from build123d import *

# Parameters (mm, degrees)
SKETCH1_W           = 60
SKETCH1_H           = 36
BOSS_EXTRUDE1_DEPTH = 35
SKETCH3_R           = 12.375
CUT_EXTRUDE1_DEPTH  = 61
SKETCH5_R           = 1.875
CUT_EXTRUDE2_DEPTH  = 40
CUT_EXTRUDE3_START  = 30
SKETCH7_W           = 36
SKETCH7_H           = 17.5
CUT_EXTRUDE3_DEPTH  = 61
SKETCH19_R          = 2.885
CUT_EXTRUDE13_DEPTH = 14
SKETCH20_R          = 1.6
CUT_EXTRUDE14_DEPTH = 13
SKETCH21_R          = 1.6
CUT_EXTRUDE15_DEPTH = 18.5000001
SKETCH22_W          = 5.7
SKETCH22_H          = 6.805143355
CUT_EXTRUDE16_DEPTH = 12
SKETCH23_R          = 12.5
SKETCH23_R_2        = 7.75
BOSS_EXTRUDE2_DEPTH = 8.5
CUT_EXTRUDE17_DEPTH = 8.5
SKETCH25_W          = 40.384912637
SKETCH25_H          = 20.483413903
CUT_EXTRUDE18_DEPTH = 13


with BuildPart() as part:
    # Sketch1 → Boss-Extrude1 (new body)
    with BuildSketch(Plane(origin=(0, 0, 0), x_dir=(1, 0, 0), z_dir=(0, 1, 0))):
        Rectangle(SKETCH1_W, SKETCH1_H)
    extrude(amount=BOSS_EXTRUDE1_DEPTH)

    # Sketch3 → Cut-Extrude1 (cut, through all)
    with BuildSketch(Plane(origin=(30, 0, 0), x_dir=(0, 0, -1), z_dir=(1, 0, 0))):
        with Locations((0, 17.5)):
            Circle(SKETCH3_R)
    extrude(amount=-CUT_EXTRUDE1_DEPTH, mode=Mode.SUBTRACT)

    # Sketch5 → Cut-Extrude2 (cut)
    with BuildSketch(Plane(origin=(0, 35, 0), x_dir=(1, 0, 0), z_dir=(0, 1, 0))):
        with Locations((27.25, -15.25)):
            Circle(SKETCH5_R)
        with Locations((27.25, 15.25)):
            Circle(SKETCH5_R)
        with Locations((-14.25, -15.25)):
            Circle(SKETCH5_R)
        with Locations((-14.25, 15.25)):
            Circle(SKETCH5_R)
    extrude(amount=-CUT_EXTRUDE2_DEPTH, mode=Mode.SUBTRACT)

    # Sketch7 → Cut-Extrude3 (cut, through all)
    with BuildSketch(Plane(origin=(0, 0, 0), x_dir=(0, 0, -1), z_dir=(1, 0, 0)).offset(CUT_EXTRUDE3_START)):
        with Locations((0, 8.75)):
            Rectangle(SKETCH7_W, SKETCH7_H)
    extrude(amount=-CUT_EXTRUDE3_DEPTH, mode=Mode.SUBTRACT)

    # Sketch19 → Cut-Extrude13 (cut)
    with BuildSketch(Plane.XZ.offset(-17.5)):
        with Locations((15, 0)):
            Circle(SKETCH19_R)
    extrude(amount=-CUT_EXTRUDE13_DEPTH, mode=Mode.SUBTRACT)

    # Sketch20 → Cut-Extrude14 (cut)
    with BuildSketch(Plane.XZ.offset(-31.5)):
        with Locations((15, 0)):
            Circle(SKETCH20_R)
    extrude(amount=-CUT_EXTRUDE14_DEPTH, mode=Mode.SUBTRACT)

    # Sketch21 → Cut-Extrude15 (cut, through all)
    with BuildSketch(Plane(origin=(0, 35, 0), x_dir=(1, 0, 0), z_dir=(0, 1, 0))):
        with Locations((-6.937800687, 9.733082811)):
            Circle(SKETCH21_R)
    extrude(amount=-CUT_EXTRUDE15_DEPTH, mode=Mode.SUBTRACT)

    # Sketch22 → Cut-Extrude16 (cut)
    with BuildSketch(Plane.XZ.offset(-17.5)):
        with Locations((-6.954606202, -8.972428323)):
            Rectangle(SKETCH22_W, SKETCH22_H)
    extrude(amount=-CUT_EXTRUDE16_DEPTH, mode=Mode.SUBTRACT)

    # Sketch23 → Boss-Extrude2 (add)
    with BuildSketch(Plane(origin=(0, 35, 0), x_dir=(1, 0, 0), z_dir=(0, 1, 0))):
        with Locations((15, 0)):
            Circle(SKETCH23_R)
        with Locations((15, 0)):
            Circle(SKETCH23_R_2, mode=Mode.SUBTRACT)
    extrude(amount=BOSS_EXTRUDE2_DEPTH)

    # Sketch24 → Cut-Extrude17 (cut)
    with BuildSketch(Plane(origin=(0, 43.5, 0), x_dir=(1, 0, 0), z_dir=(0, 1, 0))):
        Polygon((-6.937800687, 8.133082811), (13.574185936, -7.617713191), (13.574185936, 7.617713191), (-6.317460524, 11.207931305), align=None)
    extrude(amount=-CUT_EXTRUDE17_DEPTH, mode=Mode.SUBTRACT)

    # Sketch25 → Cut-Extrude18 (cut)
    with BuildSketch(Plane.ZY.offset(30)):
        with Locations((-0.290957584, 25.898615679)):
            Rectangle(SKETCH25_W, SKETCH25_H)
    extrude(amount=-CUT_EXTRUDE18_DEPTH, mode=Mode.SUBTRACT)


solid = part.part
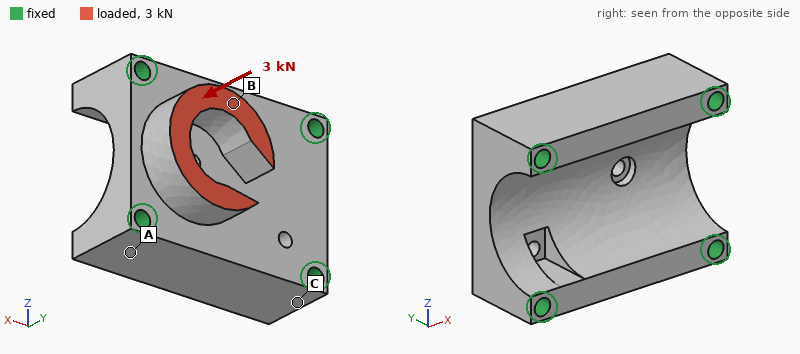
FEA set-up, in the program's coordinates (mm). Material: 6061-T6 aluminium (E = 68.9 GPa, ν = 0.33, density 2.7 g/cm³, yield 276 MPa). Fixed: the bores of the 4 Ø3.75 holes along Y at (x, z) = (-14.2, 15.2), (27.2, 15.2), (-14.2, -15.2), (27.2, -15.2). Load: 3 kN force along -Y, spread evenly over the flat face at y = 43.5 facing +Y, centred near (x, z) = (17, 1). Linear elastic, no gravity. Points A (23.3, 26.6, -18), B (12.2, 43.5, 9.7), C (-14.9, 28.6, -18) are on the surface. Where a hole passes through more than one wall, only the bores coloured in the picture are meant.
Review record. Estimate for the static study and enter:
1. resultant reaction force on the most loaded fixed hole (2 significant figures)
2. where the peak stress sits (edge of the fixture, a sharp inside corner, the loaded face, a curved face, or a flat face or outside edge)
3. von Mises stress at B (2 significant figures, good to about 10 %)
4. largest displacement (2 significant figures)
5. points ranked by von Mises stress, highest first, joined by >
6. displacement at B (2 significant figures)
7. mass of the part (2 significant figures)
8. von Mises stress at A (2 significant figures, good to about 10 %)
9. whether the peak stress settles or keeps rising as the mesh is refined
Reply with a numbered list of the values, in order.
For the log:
1. 1.3 kN
2. edge of the fixture
3. 11 MPa
4. 8.1 µm
5. B > A > C
6. 6.0 µm
7. 52 g
8. 6.0 MPa
9. keeps rising
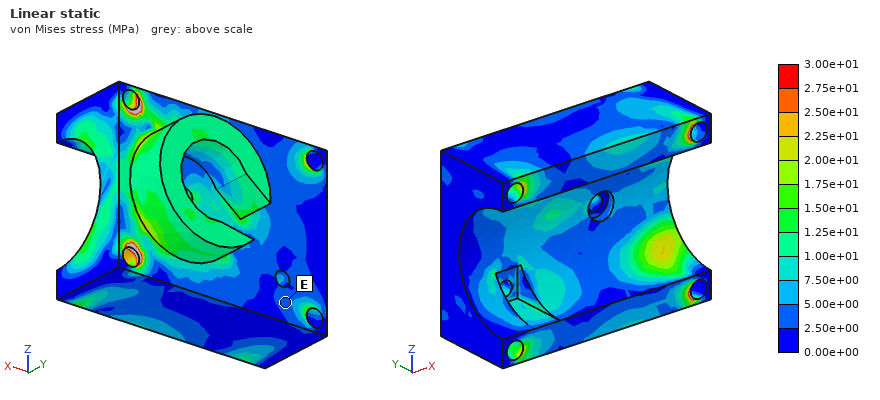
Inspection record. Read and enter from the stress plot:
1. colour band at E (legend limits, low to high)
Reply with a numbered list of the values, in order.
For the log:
1. 2.50e+00 to 5.00e+00 MPa
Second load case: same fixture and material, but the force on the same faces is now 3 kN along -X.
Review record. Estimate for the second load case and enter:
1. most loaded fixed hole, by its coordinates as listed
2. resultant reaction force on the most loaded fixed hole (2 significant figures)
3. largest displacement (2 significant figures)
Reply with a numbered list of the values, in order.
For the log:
1. (27.2, 15.2)
2. 1.2 kN
3. 29 µm
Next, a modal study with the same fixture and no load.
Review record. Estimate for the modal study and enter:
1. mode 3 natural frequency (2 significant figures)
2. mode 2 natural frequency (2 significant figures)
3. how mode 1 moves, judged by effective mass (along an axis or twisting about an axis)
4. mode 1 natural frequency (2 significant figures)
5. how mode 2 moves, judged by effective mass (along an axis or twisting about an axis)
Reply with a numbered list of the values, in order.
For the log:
1. 27 kHz
2. 25 kHz
3. along Y
4. 22 kHz
5. along Z
